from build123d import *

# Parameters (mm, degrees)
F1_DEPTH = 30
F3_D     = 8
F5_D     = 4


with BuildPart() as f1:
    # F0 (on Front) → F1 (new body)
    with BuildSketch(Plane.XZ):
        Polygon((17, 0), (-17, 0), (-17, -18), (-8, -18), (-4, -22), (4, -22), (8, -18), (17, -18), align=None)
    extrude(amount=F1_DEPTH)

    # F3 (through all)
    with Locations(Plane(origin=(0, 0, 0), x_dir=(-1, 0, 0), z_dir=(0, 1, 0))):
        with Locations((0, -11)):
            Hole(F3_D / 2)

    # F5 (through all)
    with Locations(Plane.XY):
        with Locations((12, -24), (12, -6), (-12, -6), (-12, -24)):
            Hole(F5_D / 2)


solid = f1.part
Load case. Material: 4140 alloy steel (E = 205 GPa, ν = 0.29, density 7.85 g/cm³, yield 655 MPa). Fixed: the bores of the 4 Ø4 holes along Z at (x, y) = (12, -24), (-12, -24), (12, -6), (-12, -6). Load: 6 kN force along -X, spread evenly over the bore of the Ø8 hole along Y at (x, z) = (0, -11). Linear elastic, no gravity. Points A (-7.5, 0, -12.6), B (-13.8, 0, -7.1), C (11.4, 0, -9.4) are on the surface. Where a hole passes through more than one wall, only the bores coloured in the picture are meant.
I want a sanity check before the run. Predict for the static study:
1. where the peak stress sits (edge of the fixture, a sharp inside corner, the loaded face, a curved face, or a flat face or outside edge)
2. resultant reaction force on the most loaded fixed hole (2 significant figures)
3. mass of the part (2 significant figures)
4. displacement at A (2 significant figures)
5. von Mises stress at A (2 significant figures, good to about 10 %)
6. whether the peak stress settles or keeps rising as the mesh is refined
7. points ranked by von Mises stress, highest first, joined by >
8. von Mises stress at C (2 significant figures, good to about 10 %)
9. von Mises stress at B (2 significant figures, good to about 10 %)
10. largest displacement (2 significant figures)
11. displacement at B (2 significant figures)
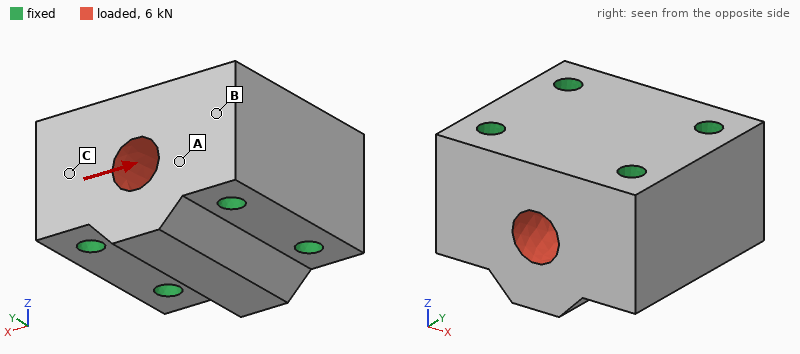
edge of the fixture
1.5 kN
140 g
0.24 µm
6.2 MPa
keeps rising
A > C > B
3.3 MPa
1.8 MPa
0.52 µm
0.091 µm
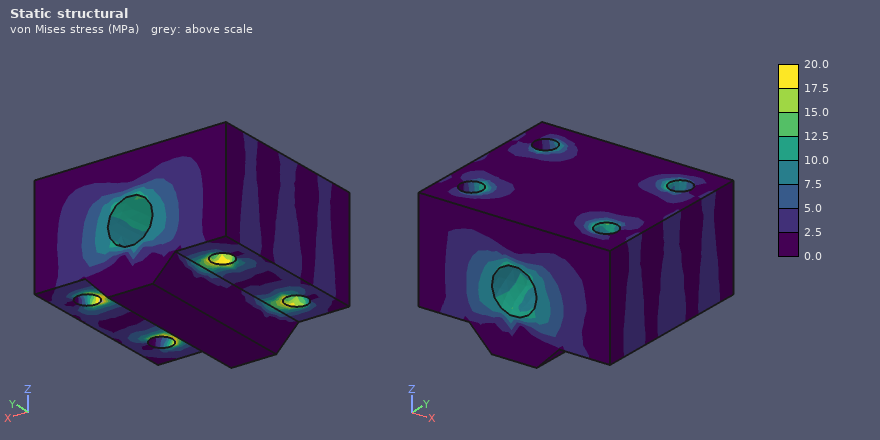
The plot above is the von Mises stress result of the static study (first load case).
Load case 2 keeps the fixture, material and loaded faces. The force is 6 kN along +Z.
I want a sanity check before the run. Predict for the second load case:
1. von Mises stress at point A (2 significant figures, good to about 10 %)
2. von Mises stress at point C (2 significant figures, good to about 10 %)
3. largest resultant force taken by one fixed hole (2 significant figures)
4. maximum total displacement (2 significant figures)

11 MPa
5.1 MPa
1.5 kN
0.97 µm
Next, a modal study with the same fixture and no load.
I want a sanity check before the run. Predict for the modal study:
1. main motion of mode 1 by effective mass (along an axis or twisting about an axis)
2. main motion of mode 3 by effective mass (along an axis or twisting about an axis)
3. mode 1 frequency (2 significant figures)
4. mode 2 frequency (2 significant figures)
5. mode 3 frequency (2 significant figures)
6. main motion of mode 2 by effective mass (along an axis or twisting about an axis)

along Y
along Y
54 kHz
58 kHz
65 kHz
along Z
